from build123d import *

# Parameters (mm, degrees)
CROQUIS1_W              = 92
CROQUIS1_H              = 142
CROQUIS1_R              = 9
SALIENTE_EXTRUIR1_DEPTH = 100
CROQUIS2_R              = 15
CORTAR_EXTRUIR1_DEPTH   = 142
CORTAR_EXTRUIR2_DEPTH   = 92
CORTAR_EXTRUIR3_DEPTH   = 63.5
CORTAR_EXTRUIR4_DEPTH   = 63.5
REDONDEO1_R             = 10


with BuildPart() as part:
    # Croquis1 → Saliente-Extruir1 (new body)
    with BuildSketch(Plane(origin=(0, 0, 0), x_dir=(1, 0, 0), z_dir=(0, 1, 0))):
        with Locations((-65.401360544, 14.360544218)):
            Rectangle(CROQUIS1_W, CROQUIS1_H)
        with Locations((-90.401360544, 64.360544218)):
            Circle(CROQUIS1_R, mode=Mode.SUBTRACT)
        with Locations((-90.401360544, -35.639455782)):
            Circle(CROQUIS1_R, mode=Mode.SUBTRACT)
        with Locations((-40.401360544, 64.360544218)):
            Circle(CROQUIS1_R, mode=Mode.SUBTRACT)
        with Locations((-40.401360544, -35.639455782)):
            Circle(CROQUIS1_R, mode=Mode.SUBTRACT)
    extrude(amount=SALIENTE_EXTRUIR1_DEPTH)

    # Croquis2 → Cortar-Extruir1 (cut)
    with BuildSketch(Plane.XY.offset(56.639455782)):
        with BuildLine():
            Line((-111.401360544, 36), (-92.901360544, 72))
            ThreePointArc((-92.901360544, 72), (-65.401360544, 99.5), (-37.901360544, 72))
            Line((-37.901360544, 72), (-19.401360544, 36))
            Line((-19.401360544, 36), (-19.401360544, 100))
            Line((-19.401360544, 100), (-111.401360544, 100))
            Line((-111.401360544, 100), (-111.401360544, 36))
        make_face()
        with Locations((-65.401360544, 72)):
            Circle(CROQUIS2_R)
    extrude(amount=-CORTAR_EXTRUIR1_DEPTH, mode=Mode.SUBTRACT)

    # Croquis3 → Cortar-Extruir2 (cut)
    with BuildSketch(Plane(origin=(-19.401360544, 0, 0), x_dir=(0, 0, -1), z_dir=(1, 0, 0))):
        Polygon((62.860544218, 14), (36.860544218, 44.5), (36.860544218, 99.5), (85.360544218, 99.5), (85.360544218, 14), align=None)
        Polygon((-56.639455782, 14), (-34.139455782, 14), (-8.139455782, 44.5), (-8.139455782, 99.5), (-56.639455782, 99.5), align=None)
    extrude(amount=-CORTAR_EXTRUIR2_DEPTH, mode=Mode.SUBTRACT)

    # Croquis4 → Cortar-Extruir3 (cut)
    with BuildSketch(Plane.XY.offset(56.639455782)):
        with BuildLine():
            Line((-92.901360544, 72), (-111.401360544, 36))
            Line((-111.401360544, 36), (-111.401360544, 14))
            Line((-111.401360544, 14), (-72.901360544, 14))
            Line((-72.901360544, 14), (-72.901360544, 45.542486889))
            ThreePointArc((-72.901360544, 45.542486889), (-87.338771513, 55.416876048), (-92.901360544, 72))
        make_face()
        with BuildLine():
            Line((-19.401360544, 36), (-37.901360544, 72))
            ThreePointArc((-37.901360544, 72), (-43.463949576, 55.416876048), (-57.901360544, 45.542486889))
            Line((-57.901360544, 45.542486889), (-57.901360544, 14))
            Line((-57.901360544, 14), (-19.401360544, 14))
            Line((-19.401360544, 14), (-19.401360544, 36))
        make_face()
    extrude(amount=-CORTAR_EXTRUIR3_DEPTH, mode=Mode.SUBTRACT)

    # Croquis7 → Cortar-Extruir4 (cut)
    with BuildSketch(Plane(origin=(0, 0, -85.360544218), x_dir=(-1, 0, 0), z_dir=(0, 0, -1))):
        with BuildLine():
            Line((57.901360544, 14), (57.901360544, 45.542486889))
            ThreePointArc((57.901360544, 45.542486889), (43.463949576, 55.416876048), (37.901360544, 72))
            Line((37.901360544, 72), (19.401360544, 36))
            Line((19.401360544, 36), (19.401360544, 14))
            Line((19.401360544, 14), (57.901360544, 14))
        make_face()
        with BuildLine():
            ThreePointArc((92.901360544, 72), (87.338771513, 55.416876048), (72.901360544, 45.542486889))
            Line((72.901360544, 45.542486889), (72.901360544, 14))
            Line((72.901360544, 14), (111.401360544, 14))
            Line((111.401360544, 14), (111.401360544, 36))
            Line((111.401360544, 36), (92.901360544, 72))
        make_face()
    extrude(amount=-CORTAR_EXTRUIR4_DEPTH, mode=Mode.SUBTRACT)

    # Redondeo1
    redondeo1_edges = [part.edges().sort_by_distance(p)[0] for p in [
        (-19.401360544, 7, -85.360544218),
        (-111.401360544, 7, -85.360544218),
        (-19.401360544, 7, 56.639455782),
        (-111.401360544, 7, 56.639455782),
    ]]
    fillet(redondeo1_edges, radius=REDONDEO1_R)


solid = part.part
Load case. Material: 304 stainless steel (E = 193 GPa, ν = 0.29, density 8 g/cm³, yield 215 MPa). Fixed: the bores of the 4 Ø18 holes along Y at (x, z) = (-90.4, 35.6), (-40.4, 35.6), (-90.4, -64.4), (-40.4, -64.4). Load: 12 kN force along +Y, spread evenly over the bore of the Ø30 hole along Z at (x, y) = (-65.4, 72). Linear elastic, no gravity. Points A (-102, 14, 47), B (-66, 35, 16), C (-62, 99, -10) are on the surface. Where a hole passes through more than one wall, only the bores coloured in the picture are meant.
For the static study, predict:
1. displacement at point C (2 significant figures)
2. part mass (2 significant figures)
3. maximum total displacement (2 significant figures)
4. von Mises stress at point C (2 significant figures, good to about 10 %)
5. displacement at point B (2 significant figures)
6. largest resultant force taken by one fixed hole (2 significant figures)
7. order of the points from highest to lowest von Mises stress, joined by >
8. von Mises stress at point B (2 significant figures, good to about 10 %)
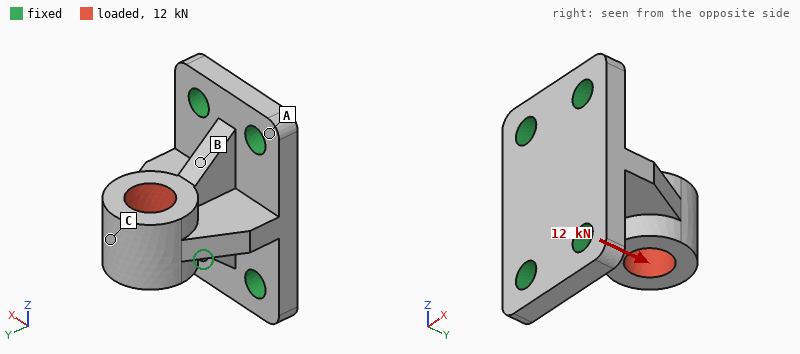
9.4 µm
2.6 kg
9.7 µm
7.3 MPa
4.2 µm
3.3 kN
B > C > A
17 MPa
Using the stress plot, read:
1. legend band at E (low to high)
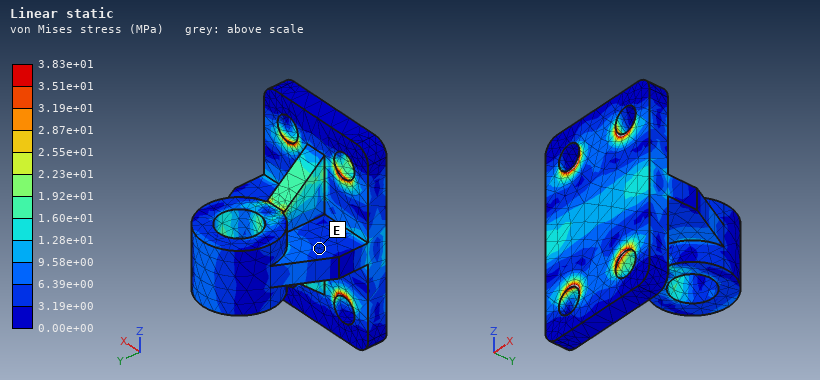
3.19e+00 to 6.39e+00 MPa
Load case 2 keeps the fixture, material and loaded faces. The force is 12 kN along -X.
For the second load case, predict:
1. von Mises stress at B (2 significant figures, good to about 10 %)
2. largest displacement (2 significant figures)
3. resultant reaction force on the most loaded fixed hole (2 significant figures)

34 MPa
84 µm
7.9 kN
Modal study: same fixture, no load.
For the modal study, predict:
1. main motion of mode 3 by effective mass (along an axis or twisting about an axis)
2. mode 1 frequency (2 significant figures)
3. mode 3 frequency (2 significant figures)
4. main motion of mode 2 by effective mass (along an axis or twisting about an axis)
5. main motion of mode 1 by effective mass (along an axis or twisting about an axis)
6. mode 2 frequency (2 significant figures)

along Y
2400 Hz
5400 Hz
along Z
along X
3500 Hz
